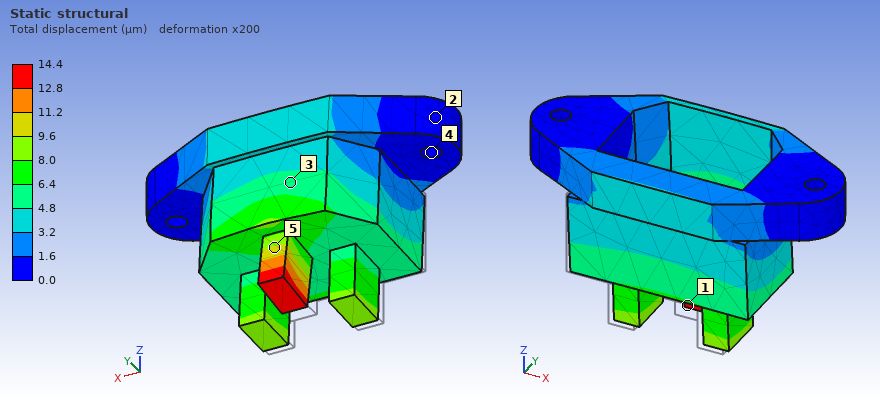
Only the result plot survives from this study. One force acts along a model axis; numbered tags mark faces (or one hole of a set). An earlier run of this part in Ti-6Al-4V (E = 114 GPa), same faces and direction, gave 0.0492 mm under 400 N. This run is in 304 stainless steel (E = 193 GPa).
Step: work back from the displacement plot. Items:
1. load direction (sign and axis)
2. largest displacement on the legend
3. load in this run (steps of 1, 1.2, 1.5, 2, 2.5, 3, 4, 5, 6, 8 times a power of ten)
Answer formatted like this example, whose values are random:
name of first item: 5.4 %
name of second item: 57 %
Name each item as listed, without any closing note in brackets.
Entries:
load direction: +Y
largest displacement on the legend: 14.4 µm
load in this run: 200 N
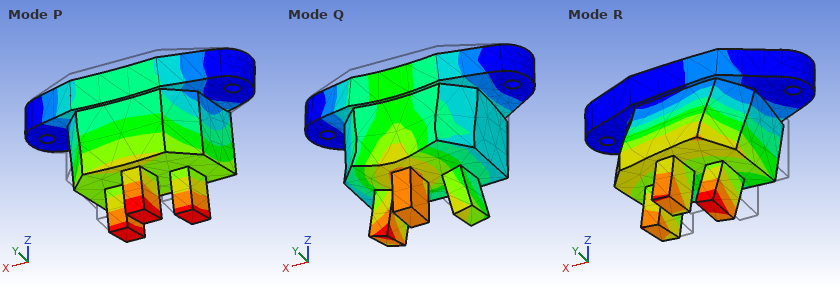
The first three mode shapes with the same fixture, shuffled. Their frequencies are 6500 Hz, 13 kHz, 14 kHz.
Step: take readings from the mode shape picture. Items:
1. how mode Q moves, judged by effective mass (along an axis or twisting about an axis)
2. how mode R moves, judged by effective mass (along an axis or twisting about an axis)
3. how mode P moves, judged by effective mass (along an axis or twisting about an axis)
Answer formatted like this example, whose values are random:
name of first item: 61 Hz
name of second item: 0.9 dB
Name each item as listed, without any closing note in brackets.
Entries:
how mode Q moves, judged by effective mass: along Z
how mode R moves, judged by effective mass: along X
how mode P moves, judged by effective mass: along Y
